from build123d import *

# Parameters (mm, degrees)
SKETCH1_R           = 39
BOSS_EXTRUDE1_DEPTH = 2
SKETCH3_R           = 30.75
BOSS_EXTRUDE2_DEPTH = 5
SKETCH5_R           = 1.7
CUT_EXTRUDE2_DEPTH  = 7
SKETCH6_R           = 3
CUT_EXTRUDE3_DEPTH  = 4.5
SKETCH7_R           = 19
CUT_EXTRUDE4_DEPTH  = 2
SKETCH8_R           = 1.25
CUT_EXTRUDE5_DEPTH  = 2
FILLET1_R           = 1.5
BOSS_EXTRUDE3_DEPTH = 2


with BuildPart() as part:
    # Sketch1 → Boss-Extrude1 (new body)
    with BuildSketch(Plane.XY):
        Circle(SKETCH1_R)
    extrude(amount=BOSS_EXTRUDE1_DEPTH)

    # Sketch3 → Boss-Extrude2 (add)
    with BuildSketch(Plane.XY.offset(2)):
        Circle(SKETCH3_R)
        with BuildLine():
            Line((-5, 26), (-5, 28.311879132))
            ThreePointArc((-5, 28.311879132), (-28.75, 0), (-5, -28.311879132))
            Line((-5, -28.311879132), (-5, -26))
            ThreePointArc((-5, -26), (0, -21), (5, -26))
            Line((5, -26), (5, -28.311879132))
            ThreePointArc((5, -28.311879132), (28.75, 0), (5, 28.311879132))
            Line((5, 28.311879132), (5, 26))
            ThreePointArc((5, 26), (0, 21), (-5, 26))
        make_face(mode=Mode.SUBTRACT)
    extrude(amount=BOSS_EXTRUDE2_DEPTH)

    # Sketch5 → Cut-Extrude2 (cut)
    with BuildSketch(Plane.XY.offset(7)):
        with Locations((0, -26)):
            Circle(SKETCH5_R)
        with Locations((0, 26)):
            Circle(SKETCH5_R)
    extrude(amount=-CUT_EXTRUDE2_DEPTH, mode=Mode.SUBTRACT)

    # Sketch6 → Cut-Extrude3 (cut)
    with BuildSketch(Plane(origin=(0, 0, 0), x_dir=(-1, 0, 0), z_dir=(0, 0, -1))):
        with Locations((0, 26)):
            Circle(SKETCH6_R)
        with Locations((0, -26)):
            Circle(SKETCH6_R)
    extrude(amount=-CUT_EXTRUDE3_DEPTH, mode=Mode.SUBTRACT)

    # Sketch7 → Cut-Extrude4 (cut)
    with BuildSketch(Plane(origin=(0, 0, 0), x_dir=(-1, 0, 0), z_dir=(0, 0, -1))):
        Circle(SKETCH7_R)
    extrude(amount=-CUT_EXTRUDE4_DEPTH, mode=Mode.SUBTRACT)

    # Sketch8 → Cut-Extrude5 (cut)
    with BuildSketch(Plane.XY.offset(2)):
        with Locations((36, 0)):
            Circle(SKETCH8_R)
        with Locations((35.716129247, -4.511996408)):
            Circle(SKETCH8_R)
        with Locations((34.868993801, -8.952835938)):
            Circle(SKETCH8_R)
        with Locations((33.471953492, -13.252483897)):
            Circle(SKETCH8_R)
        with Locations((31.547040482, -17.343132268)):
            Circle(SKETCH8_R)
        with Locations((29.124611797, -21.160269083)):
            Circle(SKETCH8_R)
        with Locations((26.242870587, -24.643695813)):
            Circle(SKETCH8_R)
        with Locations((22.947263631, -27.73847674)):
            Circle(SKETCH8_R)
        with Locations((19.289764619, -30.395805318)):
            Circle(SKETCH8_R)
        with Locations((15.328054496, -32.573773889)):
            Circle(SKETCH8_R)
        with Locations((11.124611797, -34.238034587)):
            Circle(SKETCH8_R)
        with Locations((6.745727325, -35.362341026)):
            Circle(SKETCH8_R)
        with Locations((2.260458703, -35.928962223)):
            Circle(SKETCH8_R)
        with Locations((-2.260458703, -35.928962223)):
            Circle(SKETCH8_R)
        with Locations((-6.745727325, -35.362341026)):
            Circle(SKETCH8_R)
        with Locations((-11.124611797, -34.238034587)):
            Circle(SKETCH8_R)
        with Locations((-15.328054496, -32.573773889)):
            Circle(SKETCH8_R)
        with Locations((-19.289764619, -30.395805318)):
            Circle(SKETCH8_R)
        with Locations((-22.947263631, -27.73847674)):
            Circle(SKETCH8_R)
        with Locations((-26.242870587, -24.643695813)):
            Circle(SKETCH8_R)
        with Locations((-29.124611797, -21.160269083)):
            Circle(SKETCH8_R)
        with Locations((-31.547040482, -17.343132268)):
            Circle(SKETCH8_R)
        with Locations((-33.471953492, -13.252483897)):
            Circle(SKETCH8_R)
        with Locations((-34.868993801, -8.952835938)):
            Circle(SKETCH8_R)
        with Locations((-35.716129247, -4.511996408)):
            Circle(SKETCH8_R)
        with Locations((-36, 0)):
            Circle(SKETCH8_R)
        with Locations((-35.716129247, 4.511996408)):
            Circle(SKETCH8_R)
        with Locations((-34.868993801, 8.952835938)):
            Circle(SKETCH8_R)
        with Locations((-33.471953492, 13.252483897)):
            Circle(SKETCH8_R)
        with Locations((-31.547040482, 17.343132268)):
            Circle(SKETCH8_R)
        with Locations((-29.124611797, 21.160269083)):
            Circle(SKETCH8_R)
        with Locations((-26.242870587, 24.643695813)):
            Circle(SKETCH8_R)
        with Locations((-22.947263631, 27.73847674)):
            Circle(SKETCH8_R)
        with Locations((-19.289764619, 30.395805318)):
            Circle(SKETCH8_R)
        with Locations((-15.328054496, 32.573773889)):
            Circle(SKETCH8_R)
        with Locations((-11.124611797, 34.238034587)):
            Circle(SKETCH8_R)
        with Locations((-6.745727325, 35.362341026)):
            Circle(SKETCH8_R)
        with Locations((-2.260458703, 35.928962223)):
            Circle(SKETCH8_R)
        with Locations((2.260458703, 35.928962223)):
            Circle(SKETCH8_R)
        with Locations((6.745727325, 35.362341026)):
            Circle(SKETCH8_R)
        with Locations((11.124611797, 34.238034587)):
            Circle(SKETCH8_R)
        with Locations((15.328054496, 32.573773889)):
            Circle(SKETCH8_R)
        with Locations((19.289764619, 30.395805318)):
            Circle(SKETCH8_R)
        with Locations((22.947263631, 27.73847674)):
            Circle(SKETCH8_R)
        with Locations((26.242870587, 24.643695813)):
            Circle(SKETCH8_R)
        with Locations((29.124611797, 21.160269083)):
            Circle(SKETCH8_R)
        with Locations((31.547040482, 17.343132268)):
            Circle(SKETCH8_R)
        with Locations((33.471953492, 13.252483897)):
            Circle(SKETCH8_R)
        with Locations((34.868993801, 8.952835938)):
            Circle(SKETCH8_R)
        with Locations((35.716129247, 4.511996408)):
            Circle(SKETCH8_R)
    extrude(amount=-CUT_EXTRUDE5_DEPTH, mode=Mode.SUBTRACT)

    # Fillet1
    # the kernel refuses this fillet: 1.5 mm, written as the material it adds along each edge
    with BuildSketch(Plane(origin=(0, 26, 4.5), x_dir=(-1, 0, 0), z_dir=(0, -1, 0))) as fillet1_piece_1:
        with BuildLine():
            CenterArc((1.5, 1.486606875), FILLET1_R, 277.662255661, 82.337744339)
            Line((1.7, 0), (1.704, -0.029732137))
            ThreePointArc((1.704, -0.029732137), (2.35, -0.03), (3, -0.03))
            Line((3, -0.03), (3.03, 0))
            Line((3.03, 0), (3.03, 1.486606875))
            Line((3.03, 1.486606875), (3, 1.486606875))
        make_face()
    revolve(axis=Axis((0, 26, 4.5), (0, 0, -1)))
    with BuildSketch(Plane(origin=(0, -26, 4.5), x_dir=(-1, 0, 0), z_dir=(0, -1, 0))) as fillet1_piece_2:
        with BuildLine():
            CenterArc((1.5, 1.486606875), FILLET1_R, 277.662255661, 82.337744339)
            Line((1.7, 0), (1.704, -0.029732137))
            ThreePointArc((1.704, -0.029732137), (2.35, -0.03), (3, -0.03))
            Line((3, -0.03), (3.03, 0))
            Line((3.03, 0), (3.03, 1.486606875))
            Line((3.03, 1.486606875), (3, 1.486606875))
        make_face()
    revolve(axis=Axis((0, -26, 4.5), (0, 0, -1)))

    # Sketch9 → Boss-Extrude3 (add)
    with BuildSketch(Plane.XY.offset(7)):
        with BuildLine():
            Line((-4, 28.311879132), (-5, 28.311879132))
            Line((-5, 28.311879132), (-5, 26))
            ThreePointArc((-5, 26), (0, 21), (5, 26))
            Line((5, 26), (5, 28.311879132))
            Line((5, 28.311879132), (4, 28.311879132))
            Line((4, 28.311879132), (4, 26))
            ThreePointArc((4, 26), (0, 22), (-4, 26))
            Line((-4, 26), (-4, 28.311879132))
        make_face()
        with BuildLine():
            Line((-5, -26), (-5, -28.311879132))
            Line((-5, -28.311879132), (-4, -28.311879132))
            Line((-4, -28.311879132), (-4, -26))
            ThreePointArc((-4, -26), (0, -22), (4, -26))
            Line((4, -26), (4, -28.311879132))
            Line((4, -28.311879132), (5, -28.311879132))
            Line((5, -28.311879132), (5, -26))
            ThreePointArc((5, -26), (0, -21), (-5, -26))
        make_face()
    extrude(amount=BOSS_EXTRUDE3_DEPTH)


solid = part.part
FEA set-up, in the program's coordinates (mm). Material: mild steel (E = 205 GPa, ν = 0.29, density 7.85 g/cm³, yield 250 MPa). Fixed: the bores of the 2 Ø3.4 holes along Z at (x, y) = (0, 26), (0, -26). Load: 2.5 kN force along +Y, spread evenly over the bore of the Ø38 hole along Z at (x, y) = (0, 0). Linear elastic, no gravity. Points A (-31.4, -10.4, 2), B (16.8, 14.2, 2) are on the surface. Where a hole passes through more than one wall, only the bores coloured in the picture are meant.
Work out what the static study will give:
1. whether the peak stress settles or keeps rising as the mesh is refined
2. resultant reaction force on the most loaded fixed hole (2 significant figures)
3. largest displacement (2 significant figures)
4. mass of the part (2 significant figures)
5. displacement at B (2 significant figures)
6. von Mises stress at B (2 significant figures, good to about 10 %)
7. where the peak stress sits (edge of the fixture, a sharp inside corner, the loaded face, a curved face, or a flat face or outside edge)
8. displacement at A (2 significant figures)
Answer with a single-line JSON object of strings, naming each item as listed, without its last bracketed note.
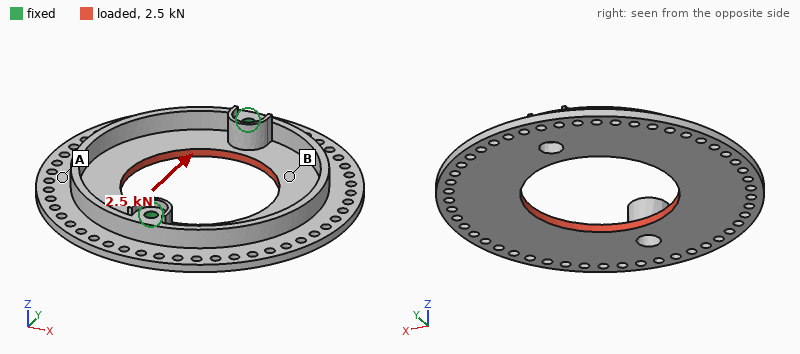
{"whether the peak stress settles or keeps rising as the mesh is refined": "keeps rising", "resultant reaction force on the most loaded fixed hole": "1.3 kN", "largest displacement": "15 µm", "mass of the part": "72 g", "displacement at B": "10.0 µm", "von Mises stress at B": "29 MPa", "where the peak stress sits": "edge of the fixture", "displacement at A": "9.5 µm"}
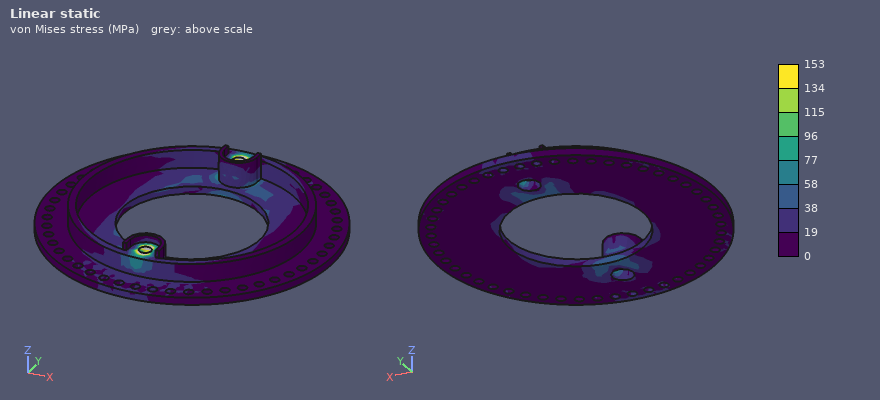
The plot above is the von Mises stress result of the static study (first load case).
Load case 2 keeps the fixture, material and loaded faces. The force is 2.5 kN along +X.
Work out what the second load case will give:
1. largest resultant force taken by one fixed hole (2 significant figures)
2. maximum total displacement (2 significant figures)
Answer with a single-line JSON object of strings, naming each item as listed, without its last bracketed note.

{"largest resultant force taken by one fixed hole": "1.3 kN", "maximum total displacement": "63 µm"}
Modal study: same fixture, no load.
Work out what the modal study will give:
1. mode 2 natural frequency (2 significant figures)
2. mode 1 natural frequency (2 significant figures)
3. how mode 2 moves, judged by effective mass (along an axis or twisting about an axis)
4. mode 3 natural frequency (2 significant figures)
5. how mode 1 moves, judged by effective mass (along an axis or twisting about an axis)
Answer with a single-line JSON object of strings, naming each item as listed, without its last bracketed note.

{"mode 2 natural frequency": "2500 Hz", "mode 1 natural frequency": "1900 Hz", "how mode 2 moves, judged by effective mass": "along Z", "mode 3 natural frequency": "4400 Hz", "how mode 1 moves, judged by effective mass": "twisting about Y"}
